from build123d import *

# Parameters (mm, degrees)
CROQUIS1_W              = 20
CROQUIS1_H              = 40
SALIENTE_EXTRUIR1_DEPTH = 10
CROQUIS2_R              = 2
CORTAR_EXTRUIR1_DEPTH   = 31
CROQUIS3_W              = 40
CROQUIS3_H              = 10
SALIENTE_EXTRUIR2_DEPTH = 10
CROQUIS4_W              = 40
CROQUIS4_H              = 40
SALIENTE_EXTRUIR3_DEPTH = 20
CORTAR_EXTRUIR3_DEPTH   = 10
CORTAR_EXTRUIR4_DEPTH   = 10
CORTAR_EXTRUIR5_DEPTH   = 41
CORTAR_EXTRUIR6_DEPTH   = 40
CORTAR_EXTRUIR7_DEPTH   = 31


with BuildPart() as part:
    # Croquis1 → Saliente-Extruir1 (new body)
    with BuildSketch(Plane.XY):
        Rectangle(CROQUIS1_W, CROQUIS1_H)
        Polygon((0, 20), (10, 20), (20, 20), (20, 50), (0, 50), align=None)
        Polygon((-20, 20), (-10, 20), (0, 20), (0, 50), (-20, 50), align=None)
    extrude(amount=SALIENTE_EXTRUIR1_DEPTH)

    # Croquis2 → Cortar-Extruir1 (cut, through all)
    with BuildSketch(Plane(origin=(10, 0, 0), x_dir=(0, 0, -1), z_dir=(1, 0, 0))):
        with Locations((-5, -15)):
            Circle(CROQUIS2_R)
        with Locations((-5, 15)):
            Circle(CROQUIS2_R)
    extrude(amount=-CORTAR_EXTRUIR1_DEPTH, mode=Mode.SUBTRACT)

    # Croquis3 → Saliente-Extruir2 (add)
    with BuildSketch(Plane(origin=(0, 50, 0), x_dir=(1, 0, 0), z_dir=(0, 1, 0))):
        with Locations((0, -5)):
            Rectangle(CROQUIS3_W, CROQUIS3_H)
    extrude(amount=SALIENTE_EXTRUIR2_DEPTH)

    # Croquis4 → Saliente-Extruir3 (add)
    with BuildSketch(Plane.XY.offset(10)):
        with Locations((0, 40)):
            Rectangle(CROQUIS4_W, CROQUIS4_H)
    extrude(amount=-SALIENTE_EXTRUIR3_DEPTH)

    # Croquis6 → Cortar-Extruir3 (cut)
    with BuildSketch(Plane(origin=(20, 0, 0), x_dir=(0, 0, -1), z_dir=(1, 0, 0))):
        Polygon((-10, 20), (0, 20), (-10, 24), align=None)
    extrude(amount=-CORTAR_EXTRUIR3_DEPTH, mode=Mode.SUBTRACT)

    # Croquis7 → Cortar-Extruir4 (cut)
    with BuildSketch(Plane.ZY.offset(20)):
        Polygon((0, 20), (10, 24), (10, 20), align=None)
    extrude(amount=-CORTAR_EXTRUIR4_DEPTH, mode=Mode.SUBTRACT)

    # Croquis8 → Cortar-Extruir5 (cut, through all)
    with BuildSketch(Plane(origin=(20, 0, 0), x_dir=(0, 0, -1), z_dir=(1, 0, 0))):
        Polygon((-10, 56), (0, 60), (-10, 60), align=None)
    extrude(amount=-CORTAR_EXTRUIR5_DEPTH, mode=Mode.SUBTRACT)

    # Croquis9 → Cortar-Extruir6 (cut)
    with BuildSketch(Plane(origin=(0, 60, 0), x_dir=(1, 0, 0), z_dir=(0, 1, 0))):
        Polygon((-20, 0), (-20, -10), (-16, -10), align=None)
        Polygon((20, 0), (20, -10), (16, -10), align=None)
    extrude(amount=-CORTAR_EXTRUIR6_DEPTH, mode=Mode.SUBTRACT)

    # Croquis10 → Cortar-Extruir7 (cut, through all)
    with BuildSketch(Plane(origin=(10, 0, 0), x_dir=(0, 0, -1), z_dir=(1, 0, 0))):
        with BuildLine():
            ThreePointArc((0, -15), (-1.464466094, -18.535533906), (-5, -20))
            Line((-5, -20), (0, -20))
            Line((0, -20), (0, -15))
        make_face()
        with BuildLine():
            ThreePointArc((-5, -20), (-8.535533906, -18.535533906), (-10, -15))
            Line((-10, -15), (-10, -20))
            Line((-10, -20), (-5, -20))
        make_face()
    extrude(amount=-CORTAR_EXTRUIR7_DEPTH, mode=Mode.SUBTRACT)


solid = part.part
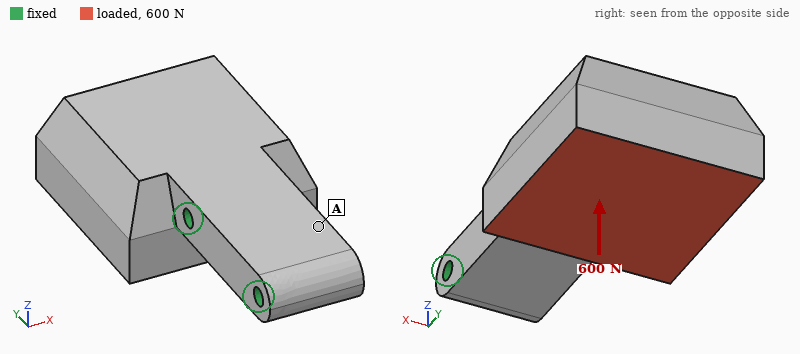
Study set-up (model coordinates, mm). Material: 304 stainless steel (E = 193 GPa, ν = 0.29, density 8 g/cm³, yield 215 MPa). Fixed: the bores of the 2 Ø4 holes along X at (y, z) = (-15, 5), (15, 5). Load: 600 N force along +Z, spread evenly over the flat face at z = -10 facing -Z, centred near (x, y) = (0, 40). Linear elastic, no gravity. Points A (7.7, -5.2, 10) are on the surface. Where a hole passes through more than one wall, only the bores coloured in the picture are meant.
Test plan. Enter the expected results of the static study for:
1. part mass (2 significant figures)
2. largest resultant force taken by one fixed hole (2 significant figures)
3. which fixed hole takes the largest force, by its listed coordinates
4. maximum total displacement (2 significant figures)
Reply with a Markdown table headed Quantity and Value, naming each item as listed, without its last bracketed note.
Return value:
| Quantity | Value |
|---|---|
| part mass | 290 g |
| largest resultant force taken by one fixed hole | 750 N |
| which fixed hole takes the largest force, by its listed coordinates | (15, 5) |
| maximum total displacement | 20 µm |
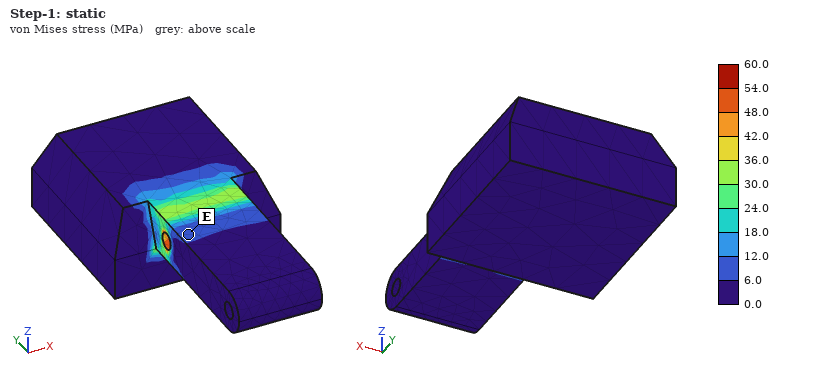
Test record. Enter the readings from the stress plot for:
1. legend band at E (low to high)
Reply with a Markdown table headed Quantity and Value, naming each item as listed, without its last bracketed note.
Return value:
| Quantity | Value |
|---|---|
| legend band at E | 6.0 to 12.0 MPa |
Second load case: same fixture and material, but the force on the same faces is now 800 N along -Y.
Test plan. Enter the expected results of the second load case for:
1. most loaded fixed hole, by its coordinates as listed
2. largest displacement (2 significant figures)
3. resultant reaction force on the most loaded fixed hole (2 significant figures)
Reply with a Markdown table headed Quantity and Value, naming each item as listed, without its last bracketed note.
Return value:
| Quantity | Value |
|---|---|
| most loaded fixed hole, by its coordinates as listed | (15, 5) |
| largest displacement | 19 µm |
| resultant reaction force on the most loaded fixed hole | 790 N |
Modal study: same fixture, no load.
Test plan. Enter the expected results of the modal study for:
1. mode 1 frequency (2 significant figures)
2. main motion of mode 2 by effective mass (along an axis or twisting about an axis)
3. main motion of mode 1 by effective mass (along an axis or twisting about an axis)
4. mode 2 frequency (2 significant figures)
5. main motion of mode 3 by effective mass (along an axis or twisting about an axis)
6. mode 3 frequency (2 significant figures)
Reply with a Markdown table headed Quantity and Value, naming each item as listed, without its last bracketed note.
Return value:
| Quantity | Value |
|---|---|
| mode 1 frequency | 2200 Hz |
| main motion of mode 2 by effective mass | along X |
| main motion of mode 1 by effective mass | along Z |
| mode 2 frequency | 4100 Hz |
| main motion of mode 3 by effective mass | twisting about Y |
| mode 3 frequency | 6100 Hz |
